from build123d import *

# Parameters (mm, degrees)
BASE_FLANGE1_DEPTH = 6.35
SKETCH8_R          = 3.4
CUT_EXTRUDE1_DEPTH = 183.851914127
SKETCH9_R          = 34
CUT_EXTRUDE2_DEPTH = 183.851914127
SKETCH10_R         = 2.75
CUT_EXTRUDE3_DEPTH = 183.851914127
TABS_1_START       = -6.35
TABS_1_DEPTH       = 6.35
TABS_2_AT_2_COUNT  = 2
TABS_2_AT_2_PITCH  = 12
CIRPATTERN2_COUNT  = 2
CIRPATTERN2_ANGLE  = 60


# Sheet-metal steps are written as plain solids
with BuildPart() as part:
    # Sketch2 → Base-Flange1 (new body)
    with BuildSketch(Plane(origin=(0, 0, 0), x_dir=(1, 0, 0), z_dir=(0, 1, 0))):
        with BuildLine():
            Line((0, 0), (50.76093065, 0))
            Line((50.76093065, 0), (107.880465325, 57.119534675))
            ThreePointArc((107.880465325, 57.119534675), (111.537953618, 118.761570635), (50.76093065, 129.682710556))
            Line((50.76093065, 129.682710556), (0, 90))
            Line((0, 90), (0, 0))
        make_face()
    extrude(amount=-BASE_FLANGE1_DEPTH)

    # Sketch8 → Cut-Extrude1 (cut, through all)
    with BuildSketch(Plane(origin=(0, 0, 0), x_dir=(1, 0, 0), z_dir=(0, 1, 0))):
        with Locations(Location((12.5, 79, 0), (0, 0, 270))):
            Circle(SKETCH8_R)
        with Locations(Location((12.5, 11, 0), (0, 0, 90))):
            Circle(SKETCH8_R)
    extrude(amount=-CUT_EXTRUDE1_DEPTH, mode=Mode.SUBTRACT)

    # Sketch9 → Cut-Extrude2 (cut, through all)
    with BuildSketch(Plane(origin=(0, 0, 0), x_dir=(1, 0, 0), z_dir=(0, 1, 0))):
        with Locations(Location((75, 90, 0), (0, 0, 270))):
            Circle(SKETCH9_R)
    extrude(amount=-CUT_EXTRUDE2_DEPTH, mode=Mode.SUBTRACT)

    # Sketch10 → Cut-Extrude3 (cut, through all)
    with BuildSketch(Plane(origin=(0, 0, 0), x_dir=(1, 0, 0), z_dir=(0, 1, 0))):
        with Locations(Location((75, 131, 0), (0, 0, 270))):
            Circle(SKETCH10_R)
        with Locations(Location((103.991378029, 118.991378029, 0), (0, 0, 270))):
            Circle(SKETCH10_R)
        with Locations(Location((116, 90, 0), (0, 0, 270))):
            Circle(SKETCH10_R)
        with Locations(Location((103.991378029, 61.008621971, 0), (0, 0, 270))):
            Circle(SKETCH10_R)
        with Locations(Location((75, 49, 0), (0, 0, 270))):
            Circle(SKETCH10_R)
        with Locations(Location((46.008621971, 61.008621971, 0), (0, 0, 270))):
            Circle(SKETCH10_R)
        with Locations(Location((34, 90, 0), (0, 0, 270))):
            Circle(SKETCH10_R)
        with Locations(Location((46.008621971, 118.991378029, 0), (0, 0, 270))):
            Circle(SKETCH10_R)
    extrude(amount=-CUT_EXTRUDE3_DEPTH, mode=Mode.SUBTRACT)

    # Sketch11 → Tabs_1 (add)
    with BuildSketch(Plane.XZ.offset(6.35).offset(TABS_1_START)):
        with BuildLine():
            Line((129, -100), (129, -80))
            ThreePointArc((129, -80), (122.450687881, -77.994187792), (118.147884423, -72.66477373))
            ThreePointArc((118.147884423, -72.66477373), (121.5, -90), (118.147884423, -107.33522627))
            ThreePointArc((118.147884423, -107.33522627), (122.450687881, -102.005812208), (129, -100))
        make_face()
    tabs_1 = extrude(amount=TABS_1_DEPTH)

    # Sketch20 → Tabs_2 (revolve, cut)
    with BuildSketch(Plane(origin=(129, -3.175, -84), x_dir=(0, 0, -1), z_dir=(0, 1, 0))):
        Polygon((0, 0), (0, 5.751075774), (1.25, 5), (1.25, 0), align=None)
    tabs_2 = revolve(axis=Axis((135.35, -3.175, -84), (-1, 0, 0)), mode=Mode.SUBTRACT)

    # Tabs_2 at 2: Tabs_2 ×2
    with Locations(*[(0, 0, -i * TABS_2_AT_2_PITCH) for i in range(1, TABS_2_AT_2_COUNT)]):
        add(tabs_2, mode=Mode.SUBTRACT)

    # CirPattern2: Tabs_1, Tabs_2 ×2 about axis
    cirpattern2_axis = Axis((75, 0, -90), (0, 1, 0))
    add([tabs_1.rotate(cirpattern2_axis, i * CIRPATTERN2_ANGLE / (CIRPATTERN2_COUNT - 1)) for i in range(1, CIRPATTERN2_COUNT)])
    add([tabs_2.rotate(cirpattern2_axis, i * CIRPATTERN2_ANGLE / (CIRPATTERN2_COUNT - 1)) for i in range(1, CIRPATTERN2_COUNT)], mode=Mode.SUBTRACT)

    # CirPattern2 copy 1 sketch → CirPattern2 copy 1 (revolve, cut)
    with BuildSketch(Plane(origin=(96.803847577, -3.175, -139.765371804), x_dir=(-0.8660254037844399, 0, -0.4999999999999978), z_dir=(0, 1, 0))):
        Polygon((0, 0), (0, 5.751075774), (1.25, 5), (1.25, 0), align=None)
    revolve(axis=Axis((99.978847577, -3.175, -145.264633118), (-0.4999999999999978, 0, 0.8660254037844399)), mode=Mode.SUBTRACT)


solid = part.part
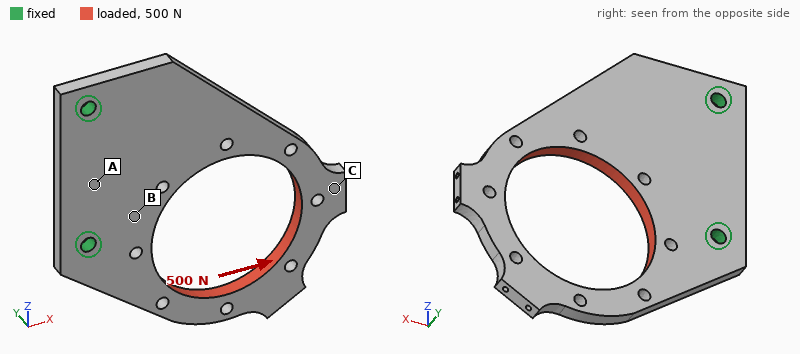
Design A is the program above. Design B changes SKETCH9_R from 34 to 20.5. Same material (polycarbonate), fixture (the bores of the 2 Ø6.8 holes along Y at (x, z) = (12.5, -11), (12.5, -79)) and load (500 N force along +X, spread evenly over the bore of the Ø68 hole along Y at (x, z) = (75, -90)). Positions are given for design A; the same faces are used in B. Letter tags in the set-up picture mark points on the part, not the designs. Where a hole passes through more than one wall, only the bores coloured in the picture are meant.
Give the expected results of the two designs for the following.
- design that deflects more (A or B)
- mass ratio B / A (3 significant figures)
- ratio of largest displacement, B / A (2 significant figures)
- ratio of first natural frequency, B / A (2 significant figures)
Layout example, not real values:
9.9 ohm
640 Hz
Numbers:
A
1.27
0.29
1.0
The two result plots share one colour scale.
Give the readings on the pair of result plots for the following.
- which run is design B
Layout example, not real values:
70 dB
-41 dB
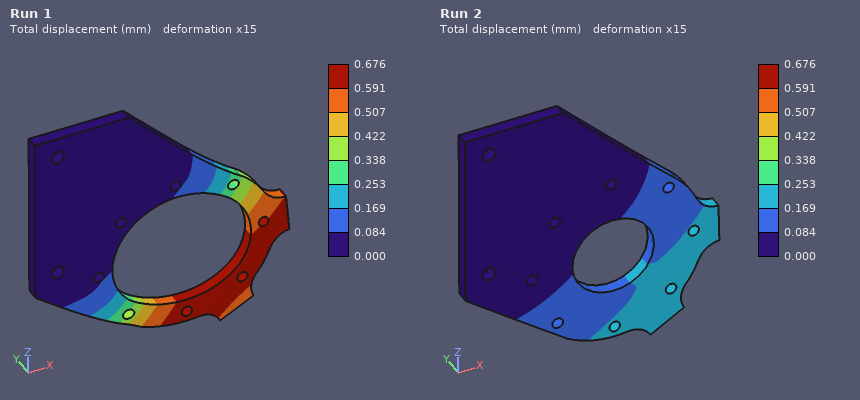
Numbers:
Run 2
